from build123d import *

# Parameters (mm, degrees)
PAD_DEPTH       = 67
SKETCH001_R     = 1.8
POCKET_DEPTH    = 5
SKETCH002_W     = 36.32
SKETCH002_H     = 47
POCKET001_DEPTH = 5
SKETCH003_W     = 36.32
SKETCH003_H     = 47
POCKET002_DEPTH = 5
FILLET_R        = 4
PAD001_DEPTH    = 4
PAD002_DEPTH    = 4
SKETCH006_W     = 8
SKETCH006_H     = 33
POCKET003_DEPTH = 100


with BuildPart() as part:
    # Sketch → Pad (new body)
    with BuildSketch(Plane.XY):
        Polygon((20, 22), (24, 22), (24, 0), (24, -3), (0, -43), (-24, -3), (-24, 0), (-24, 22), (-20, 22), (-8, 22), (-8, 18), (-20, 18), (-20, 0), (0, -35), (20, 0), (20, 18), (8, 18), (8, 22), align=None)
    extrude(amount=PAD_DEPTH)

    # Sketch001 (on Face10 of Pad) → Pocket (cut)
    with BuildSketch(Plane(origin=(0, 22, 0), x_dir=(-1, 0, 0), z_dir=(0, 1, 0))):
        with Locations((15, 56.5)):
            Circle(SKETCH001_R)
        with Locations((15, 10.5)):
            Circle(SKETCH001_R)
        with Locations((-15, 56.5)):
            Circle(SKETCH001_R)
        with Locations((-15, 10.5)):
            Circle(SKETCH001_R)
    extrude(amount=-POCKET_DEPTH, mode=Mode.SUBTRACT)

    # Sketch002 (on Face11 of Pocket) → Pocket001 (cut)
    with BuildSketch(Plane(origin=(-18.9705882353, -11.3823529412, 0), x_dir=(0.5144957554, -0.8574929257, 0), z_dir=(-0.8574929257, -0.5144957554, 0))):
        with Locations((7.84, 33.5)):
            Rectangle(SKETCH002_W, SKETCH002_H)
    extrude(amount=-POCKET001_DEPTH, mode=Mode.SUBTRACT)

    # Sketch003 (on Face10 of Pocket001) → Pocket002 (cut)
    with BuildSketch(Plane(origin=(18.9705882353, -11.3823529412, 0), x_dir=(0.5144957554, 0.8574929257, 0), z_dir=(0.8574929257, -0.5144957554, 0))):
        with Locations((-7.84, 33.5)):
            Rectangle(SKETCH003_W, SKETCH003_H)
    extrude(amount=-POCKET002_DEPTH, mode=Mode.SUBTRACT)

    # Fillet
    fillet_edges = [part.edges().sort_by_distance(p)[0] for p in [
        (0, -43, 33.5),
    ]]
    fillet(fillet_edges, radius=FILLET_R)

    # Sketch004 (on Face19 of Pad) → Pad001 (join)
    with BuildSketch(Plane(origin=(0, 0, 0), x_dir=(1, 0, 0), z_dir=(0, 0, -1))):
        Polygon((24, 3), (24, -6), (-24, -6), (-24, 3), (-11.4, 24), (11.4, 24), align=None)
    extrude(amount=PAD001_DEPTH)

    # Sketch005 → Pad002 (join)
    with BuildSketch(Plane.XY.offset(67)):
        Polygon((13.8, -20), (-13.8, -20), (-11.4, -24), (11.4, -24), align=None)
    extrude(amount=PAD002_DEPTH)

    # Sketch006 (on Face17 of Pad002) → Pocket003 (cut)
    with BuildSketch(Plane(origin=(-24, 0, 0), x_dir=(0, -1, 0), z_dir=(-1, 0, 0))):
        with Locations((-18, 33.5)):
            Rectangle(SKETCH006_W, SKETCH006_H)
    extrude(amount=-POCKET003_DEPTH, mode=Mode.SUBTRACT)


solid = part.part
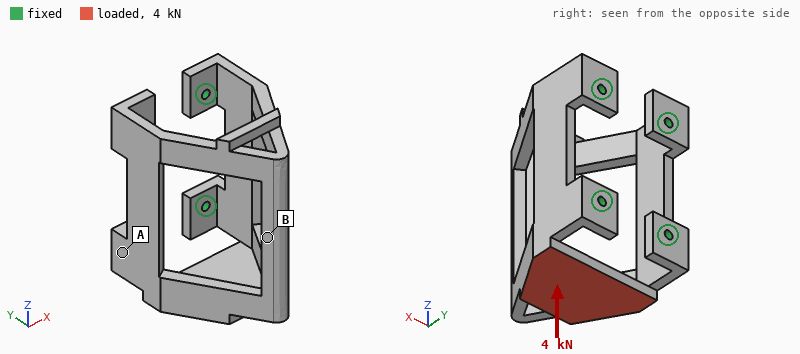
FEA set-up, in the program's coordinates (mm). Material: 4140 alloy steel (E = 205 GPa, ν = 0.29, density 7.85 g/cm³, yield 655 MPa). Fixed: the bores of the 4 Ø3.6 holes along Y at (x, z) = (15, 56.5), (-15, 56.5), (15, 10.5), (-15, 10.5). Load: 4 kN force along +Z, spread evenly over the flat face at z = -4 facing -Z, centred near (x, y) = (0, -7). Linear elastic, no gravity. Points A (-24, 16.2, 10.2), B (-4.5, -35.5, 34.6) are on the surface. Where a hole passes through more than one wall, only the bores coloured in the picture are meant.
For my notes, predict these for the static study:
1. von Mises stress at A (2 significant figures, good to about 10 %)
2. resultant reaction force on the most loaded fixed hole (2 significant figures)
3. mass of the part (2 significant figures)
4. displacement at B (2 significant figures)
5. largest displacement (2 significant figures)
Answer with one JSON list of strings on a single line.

["54 MPa", "1.5 kN", "220 g", "0.100 mm", "0.11 mm"]
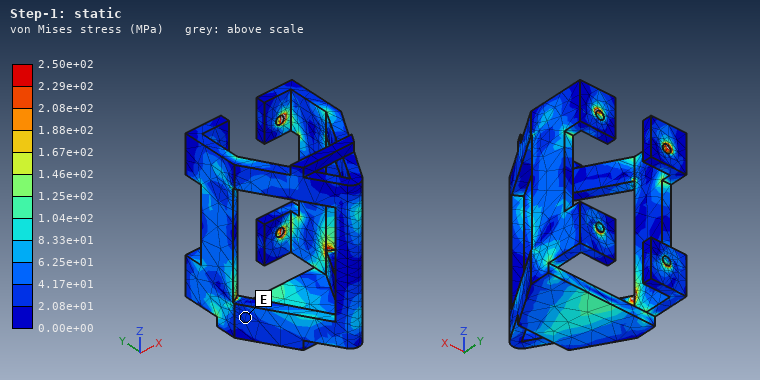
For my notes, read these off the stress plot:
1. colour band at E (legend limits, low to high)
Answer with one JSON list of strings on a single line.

["2.08e+01 to 4.17e+01 MPa"]
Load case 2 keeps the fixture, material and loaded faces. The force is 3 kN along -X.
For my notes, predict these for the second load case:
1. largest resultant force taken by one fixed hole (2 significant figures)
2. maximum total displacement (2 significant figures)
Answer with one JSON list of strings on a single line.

["1.6 kN", "0.17 mm"]
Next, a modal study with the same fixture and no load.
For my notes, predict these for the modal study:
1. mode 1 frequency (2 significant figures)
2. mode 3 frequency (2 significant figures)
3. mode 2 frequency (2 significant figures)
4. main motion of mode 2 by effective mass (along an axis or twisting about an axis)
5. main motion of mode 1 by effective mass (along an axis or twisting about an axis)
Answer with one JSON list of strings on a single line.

["1900 Hz", "2900 Hz", "2500 Hz", "along Z", "along X"]
